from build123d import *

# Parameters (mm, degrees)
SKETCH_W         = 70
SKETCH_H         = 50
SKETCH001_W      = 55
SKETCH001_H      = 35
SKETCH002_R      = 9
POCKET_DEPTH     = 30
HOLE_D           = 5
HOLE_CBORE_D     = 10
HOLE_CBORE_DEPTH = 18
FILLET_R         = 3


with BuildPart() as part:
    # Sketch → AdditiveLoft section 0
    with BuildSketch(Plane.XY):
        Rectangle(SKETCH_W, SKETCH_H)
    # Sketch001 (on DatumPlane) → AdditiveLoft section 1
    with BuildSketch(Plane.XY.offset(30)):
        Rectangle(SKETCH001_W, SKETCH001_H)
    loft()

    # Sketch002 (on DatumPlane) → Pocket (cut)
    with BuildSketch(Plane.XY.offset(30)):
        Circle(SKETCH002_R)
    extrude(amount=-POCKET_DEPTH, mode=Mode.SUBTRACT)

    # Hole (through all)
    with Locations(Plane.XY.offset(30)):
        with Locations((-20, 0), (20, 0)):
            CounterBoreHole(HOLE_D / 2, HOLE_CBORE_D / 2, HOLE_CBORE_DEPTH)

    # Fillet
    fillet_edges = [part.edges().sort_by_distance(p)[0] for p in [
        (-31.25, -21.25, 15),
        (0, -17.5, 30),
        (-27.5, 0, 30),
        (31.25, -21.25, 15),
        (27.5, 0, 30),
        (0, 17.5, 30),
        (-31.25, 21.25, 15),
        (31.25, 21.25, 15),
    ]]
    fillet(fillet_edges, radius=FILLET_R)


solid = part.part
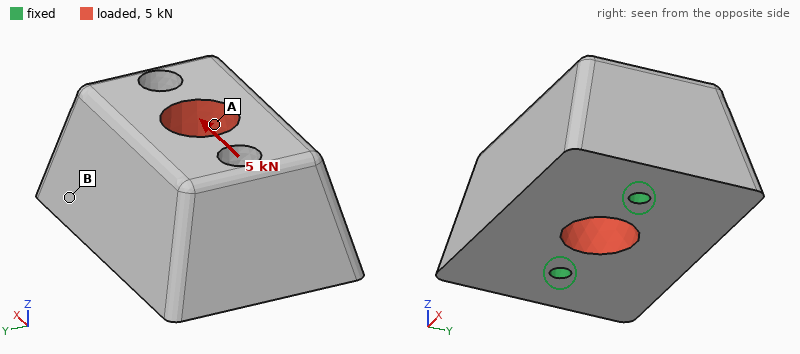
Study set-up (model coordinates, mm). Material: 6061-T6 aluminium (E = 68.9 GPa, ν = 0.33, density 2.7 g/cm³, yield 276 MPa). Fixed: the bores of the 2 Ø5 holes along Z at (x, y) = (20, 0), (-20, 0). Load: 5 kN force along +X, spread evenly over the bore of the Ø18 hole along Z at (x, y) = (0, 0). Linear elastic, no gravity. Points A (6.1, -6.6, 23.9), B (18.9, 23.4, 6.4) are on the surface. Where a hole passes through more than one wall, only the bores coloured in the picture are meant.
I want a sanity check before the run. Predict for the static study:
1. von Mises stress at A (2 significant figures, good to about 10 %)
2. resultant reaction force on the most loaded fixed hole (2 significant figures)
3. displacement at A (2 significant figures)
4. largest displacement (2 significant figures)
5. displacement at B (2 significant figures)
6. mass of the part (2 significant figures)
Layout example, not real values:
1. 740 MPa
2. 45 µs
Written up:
1. 6.0 MPa
2. 2.7 kN
3. 3.8 µm
4. 4.6 µm
5. 2.1 µm
6. 190 g
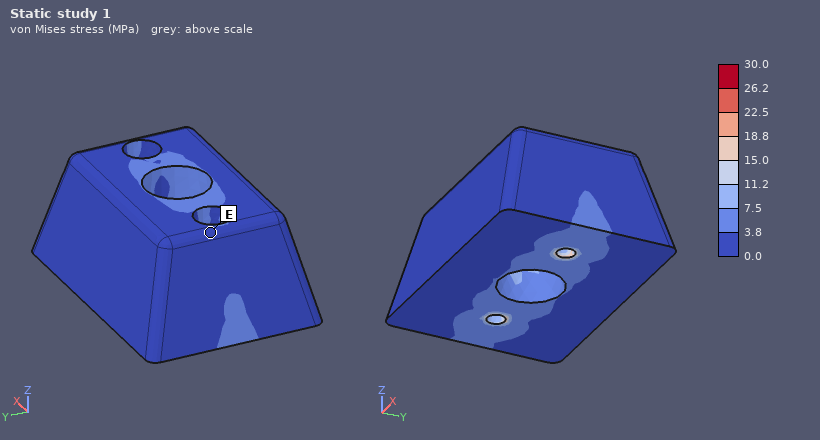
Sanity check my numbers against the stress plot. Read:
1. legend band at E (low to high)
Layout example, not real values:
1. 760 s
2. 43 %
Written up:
1. 0.0 to 3.8 MPa
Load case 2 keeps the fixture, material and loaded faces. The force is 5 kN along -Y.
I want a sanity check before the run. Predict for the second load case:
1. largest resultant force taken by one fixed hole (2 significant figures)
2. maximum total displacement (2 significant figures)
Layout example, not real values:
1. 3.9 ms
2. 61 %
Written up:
1. 2.5 kN
2. 17 µm
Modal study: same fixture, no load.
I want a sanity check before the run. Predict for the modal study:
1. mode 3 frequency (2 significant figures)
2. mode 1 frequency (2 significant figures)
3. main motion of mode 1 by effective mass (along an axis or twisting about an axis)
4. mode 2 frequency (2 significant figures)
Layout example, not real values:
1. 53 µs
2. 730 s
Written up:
1. 14 kHz
2. 6400 Hz
3. along Y
4. 14 kHz
